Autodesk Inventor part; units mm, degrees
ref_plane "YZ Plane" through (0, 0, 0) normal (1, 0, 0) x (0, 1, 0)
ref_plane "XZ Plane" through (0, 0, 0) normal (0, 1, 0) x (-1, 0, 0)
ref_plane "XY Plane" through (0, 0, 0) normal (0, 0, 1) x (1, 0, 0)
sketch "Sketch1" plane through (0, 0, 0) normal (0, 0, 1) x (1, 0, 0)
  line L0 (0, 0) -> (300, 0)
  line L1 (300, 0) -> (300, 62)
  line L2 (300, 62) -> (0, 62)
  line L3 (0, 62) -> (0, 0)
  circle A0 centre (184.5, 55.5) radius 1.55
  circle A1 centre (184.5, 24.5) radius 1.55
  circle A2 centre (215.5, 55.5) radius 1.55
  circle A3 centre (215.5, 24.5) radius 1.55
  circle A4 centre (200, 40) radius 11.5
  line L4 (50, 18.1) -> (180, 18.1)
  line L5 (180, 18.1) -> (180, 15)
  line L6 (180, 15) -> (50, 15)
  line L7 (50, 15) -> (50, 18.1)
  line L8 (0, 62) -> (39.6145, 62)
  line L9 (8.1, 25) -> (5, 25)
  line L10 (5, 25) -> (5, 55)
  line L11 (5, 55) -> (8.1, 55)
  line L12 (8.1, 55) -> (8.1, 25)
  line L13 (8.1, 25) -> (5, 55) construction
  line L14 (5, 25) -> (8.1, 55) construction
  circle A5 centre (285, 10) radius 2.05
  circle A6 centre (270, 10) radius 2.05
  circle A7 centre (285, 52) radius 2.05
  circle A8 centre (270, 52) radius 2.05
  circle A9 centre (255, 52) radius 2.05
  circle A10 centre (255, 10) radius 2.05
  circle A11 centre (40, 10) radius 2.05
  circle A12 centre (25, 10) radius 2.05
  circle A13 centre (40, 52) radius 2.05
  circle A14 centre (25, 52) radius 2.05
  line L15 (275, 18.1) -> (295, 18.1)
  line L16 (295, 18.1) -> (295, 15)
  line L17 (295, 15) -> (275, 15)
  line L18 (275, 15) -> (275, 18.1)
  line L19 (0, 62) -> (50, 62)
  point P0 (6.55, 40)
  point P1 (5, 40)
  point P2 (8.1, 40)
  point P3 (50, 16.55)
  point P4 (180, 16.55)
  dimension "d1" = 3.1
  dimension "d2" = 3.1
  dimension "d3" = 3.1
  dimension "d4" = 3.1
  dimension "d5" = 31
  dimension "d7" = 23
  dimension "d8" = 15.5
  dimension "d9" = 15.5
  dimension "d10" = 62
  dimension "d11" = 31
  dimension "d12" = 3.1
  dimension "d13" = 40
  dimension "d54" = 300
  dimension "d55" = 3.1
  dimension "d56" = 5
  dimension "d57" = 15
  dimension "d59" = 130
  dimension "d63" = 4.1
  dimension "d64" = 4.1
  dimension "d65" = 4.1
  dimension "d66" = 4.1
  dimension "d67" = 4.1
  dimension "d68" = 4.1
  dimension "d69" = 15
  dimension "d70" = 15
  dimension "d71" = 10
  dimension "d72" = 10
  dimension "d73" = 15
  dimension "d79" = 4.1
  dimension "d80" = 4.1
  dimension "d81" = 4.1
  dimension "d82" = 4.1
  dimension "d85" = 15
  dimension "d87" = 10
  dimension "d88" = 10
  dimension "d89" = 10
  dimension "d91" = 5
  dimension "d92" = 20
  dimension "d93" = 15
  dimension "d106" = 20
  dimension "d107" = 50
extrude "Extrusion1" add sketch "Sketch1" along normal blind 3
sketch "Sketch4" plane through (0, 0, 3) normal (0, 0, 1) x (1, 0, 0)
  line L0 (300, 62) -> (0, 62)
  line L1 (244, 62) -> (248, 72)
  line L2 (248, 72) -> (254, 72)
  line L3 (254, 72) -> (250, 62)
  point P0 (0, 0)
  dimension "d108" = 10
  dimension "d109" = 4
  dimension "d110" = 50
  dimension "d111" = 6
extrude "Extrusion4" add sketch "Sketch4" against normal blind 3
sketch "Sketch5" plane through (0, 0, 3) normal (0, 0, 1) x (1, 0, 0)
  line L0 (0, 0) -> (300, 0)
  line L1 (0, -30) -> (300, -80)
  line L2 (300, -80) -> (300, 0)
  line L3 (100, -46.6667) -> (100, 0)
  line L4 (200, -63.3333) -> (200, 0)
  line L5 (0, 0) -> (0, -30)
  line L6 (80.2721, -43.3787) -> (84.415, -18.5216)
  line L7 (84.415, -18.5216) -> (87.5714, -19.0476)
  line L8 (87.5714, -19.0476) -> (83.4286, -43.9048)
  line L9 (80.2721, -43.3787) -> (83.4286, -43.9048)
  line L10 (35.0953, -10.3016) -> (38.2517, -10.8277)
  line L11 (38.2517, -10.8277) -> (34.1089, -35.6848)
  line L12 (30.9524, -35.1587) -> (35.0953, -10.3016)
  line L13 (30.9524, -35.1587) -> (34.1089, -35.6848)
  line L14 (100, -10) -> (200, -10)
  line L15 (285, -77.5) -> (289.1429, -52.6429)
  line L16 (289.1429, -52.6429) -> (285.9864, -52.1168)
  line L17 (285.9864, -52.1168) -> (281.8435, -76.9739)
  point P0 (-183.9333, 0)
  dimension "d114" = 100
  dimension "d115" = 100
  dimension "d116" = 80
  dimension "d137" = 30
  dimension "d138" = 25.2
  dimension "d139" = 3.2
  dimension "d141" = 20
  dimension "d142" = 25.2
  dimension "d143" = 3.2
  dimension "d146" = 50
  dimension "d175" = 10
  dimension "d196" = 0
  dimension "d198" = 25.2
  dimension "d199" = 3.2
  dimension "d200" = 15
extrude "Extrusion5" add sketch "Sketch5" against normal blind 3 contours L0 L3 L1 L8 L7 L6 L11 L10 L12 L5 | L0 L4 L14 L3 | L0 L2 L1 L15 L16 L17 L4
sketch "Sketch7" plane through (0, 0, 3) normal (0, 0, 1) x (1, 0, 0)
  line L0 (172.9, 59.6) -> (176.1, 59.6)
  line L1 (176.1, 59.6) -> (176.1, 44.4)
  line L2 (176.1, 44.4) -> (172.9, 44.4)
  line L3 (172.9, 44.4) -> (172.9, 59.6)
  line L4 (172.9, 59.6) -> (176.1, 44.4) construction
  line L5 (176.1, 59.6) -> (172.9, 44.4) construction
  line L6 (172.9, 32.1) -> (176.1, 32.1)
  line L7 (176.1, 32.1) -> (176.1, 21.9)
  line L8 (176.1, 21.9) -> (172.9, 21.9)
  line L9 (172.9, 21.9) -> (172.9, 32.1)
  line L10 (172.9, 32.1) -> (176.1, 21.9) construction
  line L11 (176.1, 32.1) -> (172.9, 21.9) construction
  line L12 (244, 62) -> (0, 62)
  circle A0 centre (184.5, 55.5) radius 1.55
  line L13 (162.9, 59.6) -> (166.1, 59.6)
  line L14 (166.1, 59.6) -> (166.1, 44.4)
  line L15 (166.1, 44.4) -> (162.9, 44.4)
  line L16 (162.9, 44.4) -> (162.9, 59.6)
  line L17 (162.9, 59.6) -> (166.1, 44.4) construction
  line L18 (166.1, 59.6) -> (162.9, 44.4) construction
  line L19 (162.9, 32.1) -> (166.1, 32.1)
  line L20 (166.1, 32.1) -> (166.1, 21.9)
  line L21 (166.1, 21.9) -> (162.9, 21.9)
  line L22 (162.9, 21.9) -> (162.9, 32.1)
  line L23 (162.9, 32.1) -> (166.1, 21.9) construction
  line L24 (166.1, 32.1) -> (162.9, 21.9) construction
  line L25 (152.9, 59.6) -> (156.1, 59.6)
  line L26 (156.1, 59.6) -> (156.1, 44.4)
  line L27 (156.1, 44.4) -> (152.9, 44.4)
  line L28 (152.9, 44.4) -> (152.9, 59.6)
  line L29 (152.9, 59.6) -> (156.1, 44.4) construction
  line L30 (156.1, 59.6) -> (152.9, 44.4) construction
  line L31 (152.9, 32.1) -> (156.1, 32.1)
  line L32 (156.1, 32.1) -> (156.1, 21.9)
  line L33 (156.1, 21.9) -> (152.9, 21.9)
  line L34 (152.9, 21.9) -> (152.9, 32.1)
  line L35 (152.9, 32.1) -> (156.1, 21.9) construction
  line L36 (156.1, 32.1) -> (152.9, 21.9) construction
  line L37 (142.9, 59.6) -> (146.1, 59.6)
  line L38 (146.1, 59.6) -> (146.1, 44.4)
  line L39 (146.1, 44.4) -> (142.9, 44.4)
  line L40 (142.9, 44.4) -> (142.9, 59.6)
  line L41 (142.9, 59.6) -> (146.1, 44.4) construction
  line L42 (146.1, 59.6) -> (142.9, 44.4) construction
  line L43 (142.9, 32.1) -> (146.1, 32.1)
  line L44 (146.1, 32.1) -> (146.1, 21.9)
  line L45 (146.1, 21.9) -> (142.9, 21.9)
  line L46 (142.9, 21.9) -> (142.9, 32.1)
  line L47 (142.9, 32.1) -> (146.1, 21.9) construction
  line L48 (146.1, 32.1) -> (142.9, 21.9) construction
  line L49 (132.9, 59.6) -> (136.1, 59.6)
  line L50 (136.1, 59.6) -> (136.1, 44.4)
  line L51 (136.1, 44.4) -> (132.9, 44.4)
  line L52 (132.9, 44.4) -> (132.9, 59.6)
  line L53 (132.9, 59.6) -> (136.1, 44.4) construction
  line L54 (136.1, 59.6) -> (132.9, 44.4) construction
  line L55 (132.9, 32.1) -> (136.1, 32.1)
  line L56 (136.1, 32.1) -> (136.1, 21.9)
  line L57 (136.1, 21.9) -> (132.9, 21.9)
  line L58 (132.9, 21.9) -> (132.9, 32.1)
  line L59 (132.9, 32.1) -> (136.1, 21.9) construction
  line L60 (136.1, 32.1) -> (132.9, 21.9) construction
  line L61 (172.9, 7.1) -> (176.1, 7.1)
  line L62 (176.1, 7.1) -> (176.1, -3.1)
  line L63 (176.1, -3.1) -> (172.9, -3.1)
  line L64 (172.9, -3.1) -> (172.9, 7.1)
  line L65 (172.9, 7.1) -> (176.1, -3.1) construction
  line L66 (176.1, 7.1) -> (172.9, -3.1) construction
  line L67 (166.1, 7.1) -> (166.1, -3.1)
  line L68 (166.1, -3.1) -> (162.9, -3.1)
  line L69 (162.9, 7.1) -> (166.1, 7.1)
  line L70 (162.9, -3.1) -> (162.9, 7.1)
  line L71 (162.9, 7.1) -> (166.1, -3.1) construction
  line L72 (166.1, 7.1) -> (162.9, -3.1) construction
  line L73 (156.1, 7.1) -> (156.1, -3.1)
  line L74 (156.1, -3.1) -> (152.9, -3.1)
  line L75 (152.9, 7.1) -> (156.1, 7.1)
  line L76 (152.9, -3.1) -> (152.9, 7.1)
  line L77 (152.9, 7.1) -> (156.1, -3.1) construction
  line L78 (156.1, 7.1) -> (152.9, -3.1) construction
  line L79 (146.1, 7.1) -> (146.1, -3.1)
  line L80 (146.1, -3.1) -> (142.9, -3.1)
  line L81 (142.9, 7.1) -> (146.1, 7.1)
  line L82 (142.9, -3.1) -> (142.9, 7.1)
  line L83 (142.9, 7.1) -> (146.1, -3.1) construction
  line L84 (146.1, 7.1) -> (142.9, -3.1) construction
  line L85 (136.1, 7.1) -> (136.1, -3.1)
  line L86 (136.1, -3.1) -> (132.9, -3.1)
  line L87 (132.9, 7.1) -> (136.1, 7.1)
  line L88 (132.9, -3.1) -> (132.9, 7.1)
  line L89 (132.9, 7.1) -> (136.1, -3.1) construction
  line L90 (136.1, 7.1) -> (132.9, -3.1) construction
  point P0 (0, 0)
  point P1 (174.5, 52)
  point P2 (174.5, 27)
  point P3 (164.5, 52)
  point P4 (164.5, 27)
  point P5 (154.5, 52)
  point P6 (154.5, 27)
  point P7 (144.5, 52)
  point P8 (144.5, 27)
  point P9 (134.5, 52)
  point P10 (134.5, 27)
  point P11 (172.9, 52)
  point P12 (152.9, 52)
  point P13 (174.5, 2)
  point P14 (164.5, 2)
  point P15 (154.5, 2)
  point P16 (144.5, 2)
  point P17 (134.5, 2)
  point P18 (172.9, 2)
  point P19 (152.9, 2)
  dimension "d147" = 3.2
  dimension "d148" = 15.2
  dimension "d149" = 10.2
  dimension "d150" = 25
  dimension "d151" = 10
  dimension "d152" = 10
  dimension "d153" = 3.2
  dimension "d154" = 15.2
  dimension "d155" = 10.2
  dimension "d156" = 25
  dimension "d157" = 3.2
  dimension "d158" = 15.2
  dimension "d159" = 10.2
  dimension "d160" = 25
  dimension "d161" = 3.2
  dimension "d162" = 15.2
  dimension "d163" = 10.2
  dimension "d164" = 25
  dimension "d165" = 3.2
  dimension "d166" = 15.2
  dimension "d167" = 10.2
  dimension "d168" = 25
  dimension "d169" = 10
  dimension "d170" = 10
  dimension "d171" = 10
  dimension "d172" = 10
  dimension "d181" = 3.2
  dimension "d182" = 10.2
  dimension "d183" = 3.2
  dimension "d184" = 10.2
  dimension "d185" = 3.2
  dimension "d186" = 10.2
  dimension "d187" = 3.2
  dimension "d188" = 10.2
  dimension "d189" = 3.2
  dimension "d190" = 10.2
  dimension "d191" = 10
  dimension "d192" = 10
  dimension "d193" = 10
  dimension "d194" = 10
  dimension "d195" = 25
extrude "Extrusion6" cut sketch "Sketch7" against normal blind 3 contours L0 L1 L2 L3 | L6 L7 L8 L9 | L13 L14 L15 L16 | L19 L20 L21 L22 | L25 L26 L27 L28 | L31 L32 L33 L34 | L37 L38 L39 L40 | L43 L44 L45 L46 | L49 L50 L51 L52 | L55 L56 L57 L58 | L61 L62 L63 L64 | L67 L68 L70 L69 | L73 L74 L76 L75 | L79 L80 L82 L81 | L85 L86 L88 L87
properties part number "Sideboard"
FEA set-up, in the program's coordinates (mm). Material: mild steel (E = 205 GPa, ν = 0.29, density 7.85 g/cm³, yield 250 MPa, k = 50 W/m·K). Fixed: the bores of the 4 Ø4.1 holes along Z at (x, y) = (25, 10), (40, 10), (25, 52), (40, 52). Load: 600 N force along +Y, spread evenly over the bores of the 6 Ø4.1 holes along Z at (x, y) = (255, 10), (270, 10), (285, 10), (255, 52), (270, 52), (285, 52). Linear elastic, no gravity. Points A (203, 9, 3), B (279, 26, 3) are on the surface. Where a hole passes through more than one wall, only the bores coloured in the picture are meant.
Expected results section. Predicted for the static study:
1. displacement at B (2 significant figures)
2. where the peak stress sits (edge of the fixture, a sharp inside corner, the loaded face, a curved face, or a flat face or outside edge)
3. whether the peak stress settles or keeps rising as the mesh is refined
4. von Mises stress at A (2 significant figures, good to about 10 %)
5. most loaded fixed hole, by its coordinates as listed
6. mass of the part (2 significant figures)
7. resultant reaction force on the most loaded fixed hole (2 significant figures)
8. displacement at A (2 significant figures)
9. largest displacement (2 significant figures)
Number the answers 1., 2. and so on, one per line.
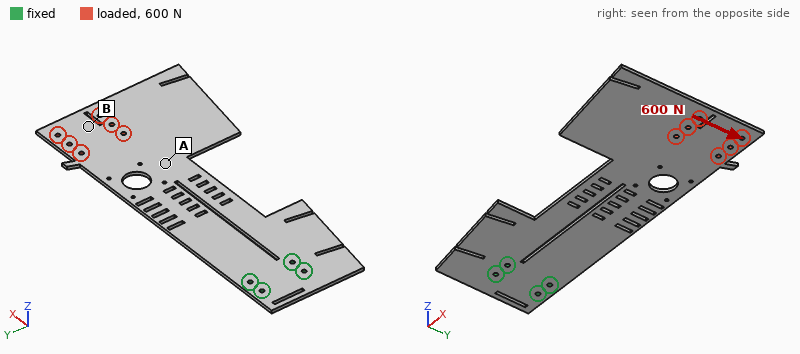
1. 0.21 mm
2. edge of the fixture
3. keeps rising
4. 14 MPa
5. (40, 52)
6. 680 g
7. 2.2 kN
8. 0.13 mm
9. 0.26 mm
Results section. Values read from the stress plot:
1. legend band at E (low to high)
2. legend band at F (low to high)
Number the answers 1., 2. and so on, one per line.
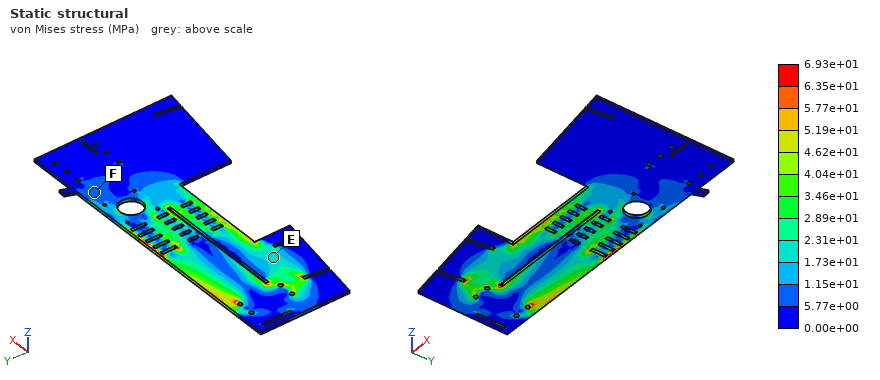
1. 1.73e+01 to 2.31e+01 MPa
2. 5.77e+00 to 1.15e+01 MPa
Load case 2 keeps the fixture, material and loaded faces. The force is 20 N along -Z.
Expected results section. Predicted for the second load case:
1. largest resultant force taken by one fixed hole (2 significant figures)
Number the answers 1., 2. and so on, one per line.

1. 99 N
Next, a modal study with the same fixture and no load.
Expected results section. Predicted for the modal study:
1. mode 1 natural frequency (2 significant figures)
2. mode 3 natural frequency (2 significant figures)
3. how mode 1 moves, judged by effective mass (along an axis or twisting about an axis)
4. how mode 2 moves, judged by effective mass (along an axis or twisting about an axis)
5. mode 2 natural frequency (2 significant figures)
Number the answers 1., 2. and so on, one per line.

1. 26 Hz
2. 190 Hz
3. along Z
4. twisting about X
5. 110 Hz
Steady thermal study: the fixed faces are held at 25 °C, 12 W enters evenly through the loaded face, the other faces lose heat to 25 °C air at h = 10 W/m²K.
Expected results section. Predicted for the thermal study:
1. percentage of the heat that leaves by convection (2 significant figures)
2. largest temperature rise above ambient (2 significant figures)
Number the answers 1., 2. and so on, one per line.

1. 95 %
2. 60 K
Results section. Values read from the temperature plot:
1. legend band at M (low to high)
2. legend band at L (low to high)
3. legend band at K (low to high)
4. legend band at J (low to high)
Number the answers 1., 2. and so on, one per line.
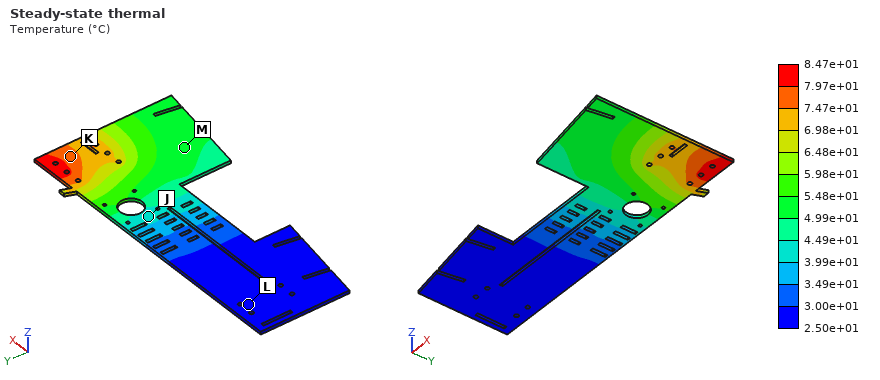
1. 4.99e+01 to 5.48e+01 °C
2. 2.50e+01 to 3.00e+01 °C
3. 7.47e+01 to 7.97e+01 °C
4. 3.99e+01 to 4.49e+01 °C
